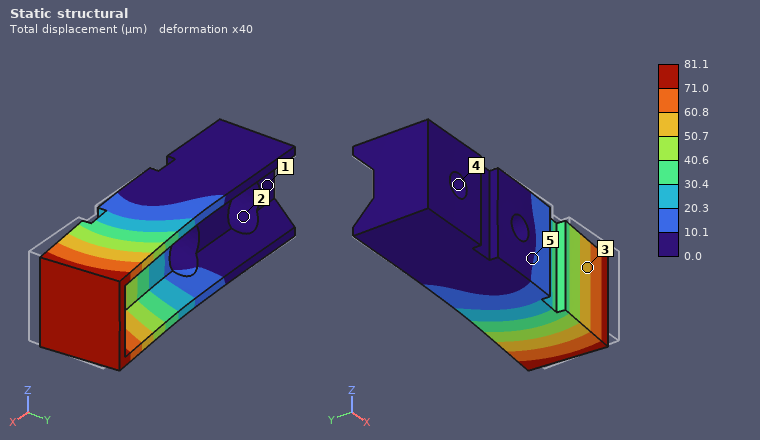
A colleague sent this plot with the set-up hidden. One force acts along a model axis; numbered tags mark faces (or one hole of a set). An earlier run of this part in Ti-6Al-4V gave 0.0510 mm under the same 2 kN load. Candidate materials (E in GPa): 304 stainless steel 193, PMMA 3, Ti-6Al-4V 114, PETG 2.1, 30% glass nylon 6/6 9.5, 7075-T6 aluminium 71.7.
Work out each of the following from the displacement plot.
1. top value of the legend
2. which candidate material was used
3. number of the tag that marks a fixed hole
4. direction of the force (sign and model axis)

81.1 µm
7075-T6 aluminium
4
+Y
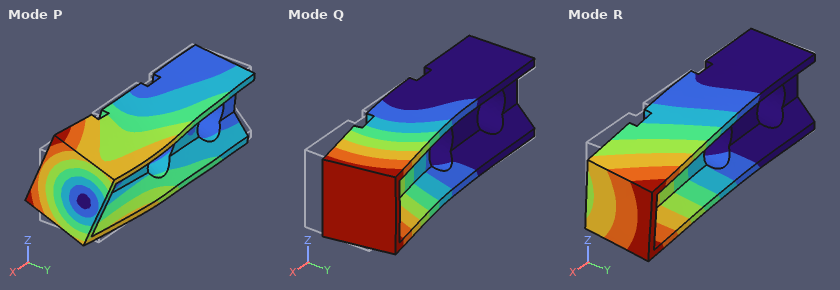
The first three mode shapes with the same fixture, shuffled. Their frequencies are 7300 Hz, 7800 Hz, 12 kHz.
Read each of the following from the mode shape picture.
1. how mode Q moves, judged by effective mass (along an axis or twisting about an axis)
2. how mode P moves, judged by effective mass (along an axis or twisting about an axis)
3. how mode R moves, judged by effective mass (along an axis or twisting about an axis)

along Y
twisting about X
along Z
